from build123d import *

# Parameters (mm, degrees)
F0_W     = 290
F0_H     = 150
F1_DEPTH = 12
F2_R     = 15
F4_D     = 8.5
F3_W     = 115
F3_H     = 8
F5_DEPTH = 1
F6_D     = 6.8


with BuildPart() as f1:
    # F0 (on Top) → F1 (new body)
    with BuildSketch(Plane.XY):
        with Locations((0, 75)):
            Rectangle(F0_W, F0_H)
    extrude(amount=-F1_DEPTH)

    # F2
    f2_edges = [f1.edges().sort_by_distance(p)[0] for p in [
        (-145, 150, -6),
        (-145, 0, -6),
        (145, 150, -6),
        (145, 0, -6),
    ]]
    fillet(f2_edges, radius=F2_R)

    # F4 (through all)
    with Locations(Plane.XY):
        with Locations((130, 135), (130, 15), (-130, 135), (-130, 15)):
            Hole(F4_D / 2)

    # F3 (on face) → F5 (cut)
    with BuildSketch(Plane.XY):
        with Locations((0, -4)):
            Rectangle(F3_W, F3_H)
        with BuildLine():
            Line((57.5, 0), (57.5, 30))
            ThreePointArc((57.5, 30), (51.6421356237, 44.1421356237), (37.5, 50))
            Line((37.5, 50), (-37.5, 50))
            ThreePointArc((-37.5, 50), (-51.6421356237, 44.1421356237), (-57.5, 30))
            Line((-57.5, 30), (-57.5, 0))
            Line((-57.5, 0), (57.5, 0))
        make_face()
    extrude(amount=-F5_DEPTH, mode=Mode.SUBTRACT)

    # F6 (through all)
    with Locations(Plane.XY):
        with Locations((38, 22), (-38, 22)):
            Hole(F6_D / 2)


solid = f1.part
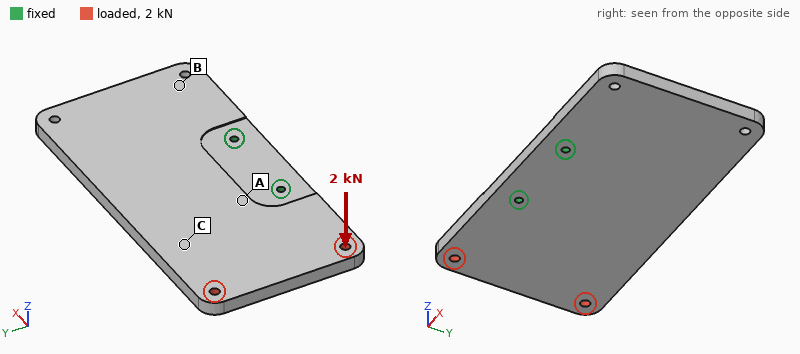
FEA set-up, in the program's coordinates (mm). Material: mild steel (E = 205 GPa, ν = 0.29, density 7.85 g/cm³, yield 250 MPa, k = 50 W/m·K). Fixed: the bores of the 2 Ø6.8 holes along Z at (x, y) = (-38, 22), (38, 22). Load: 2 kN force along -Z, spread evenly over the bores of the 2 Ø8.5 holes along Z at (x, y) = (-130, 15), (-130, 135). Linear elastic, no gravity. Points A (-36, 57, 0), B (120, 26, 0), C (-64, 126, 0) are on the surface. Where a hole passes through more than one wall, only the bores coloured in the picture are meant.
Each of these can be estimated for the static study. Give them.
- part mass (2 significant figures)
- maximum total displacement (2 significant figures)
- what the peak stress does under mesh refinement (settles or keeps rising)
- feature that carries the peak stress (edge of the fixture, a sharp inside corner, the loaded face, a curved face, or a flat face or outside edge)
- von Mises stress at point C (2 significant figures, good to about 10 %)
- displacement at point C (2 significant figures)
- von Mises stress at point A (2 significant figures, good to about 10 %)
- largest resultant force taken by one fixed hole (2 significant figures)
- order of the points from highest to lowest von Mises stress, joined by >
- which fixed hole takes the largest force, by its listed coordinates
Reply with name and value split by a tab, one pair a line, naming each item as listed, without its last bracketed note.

part mass	4.0 kg
maximum total displacement	0.47 mm
what the peak stress does under mesh refinement	keeps rising
feature that carries the peak stress	edge of the fixture
von Mises stress at point C	27 MPa
displacement at point C	0.19 mm
von Mises stress at point A	50 MPa
largest resultant force taken by one fixed hole	3.3 kN
order of the points from highest to lowest von Mises stress, joined by >	A > C > B
which fixed hole takes the largest force, by its listed coordinates	(-38, 22)
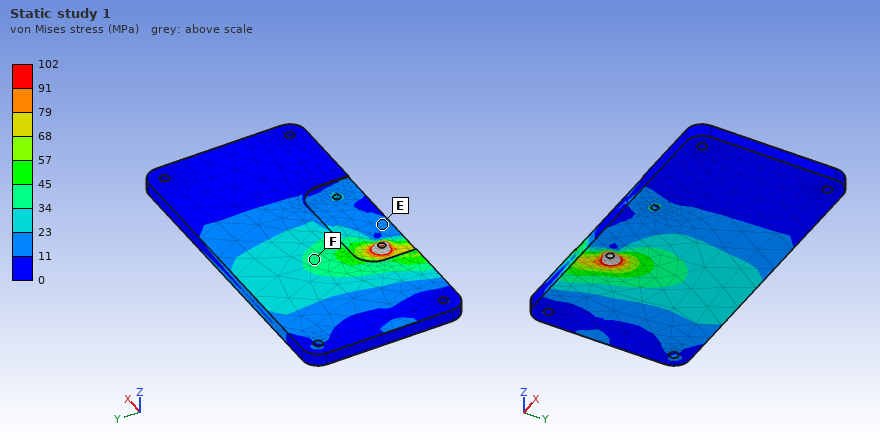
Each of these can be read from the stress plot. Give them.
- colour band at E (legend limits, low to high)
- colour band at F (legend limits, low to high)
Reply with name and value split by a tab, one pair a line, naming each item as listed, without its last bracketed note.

colour band at E	11 to 23 MPa
colour band at F	34 to 45 MPa
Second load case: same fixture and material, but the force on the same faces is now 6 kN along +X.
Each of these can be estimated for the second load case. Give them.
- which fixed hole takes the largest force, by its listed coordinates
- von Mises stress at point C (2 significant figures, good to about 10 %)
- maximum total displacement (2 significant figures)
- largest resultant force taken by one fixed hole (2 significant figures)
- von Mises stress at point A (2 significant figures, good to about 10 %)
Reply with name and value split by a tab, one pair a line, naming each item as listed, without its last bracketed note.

which fixed hole takes the largest force, by its listed coordinates	(-38, 22)
von Mises stress at point C	4.2 MPa
maximum total displacement	16 µm
largest resultant force taken by one fixed hole	5.5 kN
von Mises stress at point A	6.0 MPa
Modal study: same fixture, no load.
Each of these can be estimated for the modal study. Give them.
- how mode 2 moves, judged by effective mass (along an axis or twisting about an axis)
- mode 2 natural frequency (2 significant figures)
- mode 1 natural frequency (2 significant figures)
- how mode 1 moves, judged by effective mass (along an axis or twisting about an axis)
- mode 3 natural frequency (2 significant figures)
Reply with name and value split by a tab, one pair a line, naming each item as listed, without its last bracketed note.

how mode 2 moves, judged by effective mass	twisting about Y
mode 2 natural frequency	450 Hz
mode 1 natural frequency	380 Hz
how mode 1 moves, judged by effective mass	along Z
mode 3 natural frequency	760 Hz
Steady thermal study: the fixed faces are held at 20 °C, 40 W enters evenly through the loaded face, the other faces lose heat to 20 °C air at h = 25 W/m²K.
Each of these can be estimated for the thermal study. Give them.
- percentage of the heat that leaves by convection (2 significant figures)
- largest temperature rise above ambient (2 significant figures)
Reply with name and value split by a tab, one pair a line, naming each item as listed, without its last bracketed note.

percentage of the heat that leaves by convection	65 %
largest temperature rise above ambient	49 K
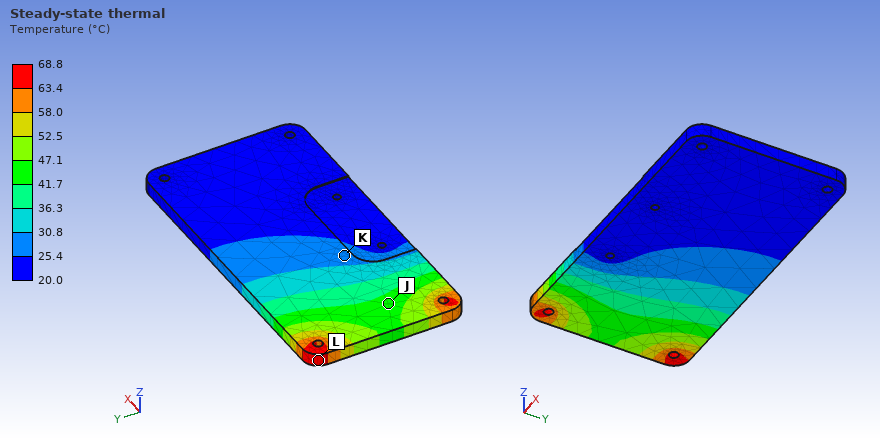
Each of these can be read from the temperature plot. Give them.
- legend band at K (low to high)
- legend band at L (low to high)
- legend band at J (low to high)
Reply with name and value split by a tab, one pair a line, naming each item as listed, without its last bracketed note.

legend band at K	25.4 to 30.8 °C
legend band at L	63.4 to 68.8 °C
legend band at J	41.7 to 47.1 °C
